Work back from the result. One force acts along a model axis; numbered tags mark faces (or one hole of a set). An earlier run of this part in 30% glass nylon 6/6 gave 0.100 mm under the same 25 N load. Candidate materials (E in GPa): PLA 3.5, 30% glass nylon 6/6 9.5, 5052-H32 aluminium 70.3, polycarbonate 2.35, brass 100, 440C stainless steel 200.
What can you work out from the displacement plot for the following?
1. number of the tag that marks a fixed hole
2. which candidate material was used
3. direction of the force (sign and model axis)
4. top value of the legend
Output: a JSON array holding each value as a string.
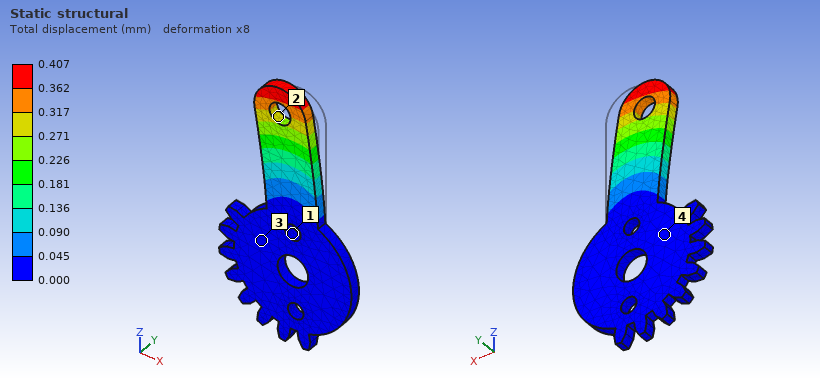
["1", "polycarbonate", "-X", "0.407 mm"]
